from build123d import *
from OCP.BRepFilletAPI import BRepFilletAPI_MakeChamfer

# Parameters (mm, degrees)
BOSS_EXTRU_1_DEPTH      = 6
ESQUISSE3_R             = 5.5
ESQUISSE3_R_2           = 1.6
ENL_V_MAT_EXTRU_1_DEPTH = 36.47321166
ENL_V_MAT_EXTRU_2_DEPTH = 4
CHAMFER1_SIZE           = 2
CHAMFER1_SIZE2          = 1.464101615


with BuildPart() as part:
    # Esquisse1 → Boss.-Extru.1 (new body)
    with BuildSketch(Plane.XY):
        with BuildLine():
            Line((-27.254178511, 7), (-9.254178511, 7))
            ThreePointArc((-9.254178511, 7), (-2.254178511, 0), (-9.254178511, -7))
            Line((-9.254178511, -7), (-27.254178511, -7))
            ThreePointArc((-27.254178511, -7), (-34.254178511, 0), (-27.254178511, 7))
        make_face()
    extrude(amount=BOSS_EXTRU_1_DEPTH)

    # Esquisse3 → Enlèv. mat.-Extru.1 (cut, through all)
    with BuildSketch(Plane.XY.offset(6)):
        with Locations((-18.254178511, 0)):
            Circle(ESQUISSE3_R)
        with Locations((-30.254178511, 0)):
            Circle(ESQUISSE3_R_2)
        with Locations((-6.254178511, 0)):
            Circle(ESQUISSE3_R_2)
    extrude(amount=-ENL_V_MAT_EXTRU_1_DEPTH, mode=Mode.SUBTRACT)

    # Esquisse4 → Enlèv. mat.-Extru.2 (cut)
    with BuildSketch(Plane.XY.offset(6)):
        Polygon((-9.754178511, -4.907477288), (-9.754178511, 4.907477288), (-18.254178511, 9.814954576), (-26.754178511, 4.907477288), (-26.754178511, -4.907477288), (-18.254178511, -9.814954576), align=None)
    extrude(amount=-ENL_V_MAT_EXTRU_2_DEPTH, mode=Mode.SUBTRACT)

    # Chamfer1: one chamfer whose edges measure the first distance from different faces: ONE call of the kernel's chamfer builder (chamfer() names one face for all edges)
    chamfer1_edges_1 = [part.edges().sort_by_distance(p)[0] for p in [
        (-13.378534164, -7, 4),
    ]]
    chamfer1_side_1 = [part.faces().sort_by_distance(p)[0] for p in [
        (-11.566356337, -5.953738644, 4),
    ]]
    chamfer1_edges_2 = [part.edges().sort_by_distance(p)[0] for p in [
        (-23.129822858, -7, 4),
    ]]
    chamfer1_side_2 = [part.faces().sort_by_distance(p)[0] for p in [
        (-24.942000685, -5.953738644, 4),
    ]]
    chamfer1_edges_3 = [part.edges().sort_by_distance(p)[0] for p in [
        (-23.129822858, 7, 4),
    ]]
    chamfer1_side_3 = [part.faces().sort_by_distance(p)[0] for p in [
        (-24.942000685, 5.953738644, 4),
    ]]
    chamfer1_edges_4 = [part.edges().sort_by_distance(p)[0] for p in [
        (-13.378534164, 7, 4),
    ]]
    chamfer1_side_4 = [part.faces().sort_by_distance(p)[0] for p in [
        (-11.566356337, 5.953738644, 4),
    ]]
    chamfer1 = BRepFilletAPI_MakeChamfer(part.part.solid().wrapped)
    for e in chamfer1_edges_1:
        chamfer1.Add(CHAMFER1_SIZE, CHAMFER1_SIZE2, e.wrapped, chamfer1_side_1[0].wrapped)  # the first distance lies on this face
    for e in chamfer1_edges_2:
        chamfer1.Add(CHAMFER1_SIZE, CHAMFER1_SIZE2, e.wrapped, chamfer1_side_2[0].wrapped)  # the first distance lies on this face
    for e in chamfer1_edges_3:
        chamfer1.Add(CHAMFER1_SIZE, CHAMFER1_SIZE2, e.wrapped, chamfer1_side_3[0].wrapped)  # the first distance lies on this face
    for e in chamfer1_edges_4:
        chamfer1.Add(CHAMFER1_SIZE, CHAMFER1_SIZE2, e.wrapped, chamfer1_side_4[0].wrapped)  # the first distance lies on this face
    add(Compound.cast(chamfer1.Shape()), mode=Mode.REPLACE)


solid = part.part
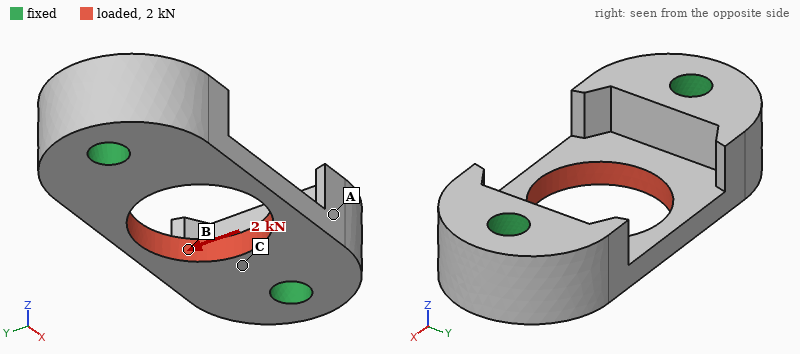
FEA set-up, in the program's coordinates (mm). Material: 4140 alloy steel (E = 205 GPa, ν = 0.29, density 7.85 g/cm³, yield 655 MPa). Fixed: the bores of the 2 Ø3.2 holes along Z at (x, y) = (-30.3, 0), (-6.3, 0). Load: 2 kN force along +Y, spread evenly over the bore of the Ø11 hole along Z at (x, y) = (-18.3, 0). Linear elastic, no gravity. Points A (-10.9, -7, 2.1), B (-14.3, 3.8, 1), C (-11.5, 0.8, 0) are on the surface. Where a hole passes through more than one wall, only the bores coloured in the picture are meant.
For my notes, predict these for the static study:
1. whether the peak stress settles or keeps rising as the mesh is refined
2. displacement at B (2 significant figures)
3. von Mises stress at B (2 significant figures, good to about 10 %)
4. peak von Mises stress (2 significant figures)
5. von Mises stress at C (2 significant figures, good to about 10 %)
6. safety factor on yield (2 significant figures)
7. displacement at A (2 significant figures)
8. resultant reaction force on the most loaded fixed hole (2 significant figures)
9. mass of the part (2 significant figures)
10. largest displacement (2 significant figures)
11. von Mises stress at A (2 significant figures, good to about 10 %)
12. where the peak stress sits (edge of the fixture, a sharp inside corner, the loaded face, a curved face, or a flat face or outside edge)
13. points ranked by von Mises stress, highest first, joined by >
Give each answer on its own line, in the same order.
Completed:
settles
6.1 µm
160 MPa
230 MPa
90 MPa
2.8
3.5 µm
1.0 kN
9.8 g
11 µm
36 MPa
a flat face or outside edge
B > C > A
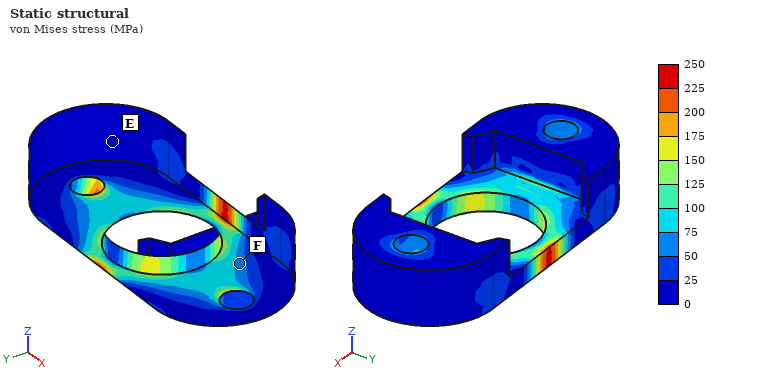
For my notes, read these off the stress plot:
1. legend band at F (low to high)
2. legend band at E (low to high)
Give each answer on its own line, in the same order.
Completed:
50 to 75 MPa
0 to 25 MPa
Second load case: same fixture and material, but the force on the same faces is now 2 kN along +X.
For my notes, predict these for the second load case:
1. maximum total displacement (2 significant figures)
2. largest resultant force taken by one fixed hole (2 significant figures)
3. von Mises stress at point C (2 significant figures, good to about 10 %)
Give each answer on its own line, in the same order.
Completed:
3.2 µm
1.0 kN
39 MPa
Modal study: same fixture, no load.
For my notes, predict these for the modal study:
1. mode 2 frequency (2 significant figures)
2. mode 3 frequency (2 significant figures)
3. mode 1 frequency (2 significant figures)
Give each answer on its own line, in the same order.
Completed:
39 kHz
56 kHz
39 kHz
